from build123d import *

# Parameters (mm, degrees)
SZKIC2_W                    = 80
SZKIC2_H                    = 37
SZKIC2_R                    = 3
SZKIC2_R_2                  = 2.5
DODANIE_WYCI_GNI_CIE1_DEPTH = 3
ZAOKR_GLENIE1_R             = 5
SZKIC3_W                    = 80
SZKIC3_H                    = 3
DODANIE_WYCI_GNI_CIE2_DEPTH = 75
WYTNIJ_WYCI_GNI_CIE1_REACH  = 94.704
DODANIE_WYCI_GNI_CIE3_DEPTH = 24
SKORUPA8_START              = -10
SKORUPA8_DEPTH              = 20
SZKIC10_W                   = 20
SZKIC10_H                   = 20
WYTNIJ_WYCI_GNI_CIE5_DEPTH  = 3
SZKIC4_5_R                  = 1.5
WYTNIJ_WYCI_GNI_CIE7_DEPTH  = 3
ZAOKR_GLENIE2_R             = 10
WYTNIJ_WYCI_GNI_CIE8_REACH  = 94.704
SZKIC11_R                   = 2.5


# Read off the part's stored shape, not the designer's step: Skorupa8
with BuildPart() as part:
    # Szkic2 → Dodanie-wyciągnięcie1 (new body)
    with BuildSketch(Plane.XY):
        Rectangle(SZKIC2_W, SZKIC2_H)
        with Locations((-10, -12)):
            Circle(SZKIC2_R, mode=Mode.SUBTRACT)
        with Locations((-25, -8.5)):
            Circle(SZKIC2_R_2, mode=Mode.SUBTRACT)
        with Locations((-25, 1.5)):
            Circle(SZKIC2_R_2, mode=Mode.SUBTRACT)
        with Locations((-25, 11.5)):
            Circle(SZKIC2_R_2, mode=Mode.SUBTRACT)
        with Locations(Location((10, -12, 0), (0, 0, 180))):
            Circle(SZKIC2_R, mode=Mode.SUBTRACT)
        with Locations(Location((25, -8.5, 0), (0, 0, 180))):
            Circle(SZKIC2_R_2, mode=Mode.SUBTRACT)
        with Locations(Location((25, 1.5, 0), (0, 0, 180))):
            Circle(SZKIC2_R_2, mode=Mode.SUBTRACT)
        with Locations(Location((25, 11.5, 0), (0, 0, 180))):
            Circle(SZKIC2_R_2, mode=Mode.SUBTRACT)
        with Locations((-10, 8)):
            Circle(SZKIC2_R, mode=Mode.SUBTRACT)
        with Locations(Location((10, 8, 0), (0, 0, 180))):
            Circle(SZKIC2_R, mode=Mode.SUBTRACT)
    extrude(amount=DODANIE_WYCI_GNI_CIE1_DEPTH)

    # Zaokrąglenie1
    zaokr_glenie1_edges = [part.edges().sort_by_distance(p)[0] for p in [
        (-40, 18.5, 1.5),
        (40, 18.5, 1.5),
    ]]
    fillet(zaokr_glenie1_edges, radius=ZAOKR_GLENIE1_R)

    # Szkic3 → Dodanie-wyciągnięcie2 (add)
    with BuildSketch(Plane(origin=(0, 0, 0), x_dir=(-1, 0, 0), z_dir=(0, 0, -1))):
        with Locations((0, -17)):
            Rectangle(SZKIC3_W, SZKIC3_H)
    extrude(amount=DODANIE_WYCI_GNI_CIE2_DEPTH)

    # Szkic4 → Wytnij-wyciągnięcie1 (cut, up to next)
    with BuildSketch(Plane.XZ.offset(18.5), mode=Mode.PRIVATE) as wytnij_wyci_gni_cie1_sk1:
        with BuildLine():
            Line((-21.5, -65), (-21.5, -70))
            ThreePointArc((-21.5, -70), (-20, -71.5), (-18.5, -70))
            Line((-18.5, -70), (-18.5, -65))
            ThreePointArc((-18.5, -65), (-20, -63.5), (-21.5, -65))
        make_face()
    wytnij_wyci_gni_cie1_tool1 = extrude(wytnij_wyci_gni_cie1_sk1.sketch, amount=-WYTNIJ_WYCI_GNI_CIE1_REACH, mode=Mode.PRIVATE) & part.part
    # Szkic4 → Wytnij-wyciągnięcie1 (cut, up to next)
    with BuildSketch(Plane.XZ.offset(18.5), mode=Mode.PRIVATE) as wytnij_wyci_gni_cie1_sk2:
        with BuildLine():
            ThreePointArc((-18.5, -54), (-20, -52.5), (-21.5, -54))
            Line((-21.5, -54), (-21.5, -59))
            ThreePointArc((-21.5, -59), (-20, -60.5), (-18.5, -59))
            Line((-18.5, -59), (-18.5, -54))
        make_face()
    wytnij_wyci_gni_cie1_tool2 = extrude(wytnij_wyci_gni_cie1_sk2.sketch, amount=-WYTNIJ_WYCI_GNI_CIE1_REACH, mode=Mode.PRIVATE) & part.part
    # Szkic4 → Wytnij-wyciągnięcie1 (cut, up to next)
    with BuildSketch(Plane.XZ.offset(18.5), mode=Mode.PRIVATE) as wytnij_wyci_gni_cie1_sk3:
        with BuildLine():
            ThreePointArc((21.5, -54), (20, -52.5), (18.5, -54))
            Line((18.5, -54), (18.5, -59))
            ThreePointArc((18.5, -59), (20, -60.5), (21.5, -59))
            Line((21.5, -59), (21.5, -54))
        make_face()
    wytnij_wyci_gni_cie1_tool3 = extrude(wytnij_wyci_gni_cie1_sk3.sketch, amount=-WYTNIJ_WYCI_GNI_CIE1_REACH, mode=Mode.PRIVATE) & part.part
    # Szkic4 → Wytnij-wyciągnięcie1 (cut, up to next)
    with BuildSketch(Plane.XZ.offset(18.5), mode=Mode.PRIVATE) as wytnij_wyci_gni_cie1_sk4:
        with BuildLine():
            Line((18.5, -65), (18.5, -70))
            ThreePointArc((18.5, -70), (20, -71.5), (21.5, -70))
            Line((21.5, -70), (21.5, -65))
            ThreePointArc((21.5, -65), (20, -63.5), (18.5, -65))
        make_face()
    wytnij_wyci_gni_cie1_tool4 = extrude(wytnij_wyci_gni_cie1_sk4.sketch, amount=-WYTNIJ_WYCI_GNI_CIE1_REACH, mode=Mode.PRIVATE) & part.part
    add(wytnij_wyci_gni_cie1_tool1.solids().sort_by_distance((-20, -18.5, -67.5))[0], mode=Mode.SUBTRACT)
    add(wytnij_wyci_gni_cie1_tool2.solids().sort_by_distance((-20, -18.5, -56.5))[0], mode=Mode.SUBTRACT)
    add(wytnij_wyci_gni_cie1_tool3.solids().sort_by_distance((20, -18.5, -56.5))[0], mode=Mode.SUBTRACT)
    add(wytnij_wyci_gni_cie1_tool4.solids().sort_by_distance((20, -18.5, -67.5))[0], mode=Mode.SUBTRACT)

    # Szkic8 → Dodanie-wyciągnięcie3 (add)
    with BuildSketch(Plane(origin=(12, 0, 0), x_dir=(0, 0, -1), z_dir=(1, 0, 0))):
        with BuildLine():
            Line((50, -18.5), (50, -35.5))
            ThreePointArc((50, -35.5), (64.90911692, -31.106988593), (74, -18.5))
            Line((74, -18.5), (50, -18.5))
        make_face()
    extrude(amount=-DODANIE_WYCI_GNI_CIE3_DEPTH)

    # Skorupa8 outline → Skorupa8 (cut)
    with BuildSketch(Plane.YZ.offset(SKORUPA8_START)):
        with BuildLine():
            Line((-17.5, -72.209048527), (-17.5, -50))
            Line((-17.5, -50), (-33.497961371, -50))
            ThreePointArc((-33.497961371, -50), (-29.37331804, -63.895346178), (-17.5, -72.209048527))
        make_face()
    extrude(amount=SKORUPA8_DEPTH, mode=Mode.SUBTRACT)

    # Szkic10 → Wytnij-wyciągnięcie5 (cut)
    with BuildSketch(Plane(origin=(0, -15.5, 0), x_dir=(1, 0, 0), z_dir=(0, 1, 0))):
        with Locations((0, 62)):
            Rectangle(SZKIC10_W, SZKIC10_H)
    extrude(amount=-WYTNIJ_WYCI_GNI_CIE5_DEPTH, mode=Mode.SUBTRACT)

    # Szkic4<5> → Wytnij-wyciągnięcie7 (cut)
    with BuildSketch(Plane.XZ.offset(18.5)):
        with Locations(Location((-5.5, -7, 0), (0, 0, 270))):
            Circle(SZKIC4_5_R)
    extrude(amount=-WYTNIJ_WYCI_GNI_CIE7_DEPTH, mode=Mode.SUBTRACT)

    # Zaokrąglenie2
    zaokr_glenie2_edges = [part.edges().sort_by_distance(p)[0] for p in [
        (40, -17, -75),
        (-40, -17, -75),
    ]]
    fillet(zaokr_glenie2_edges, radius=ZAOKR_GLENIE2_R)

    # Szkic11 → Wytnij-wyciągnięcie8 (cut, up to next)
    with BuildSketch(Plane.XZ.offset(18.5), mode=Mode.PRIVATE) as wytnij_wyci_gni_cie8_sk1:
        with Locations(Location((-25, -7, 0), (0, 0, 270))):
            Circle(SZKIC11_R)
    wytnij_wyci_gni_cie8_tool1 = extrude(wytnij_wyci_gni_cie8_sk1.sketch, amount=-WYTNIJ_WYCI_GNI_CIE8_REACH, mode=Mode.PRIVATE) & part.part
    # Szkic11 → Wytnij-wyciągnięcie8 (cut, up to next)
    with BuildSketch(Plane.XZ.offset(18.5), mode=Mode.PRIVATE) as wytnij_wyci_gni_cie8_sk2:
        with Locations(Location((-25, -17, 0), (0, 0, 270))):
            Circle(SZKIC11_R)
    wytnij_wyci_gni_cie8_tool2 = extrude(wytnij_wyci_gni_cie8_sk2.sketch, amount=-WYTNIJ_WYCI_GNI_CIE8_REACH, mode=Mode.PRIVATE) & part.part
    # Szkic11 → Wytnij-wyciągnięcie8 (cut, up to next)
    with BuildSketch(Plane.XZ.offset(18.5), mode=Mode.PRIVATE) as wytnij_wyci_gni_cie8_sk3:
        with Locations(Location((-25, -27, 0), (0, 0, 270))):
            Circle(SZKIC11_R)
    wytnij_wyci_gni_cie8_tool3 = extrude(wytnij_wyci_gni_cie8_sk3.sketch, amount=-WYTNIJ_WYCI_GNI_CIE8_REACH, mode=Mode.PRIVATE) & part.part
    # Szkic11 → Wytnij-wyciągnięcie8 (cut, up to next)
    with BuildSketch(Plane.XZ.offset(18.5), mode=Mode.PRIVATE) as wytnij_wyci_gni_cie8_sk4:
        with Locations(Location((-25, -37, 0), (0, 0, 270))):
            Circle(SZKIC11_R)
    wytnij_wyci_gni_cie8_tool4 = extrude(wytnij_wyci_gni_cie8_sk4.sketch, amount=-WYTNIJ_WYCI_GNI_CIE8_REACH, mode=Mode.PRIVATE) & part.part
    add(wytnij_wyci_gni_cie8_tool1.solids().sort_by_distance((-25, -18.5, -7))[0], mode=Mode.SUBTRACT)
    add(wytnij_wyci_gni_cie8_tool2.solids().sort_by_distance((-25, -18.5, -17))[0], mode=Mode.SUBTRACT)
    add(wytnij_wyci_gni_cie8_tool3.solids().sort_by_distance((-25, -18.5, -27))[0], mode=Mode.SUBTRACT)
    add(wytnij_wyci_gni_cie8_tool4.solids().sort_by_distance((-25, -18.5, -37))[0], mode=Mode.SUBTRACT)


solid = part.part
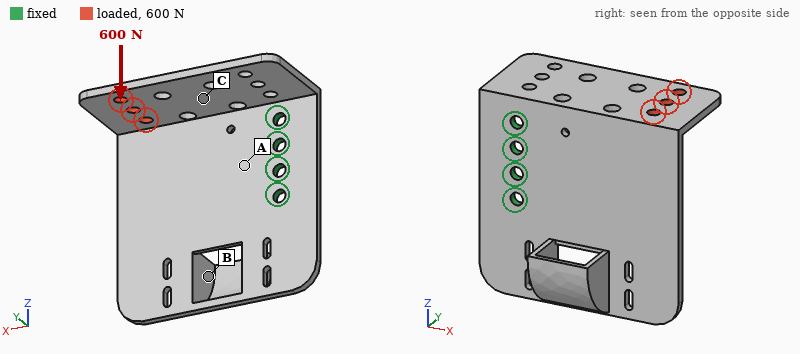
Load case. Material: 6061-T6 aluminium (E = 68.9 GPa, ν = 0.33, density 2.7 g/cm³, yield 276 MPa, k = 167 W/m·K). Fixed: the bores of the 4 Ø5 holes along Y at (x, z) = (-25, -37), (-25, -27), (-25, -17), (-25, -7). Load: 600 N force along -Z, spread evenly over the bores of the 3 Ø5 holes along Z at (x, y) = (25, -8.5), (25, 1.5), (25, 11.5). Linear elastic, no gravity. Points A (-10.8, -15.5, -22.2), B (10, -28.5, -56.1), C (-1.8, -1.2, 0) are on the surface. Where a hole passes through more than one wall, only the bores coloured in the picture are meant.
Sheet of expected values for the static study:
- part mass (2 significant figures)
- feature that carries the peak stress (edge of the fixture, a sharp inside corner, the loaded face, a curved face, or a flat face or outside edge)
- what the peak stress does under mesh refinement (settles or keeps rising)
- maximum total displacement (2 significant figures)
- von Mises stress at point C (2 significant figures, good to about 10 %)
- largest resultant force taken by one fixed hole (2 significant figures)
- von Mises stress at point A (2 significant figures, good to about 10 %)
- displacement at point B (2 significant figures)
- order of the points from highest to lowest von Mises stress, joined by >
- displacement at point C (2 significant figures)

72 g
edge of the fixture
keeps rising
1.5 mm
75 MPa
920 N
46 MPa
0.28 mm
C > A > B
0.36 mm
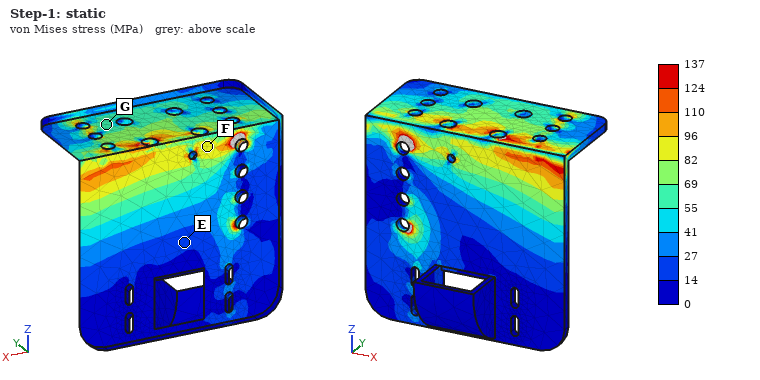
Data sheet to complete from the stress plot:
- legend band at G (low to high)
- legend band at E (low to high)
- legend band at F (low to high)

55 to 69 MPa
14 to 27 MPa
82 to 96 MPa
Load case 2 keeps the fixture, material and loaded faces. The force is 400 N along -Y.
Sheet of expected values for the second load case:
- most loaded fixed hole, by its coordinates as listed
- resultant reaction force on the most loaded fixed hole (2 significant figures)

(-25, -7)
380 N
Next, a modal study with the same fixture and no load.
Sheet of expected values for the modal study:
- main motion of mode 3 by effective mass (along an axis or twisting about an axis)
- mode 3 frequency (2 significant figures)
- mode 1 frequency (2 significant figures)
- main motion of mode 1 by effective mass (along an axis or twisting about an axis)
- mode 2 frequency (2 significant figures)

along Z
1300 Hz
640 Hz
along Y
860 Hz
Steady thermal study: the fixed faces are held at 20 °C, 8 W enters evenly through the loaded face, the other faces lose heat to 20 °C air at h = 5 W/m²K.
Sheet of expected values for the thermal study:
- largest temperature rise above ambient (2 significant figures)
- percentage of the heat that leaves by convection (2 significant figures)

18 K
6.9 %
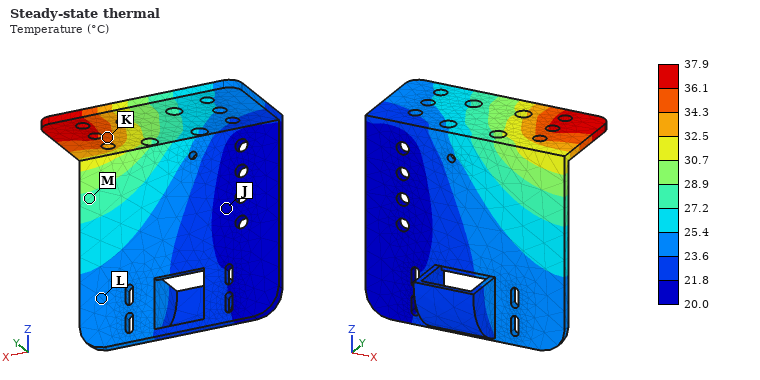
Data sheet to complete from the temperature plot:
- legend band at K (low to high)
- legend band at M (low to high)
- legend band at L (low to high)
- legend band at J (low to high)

34.3 to 36.1 °C
27.2 to 28.9 °C
23.6 to 25.4 °C
20.0 to 21.8 °C
